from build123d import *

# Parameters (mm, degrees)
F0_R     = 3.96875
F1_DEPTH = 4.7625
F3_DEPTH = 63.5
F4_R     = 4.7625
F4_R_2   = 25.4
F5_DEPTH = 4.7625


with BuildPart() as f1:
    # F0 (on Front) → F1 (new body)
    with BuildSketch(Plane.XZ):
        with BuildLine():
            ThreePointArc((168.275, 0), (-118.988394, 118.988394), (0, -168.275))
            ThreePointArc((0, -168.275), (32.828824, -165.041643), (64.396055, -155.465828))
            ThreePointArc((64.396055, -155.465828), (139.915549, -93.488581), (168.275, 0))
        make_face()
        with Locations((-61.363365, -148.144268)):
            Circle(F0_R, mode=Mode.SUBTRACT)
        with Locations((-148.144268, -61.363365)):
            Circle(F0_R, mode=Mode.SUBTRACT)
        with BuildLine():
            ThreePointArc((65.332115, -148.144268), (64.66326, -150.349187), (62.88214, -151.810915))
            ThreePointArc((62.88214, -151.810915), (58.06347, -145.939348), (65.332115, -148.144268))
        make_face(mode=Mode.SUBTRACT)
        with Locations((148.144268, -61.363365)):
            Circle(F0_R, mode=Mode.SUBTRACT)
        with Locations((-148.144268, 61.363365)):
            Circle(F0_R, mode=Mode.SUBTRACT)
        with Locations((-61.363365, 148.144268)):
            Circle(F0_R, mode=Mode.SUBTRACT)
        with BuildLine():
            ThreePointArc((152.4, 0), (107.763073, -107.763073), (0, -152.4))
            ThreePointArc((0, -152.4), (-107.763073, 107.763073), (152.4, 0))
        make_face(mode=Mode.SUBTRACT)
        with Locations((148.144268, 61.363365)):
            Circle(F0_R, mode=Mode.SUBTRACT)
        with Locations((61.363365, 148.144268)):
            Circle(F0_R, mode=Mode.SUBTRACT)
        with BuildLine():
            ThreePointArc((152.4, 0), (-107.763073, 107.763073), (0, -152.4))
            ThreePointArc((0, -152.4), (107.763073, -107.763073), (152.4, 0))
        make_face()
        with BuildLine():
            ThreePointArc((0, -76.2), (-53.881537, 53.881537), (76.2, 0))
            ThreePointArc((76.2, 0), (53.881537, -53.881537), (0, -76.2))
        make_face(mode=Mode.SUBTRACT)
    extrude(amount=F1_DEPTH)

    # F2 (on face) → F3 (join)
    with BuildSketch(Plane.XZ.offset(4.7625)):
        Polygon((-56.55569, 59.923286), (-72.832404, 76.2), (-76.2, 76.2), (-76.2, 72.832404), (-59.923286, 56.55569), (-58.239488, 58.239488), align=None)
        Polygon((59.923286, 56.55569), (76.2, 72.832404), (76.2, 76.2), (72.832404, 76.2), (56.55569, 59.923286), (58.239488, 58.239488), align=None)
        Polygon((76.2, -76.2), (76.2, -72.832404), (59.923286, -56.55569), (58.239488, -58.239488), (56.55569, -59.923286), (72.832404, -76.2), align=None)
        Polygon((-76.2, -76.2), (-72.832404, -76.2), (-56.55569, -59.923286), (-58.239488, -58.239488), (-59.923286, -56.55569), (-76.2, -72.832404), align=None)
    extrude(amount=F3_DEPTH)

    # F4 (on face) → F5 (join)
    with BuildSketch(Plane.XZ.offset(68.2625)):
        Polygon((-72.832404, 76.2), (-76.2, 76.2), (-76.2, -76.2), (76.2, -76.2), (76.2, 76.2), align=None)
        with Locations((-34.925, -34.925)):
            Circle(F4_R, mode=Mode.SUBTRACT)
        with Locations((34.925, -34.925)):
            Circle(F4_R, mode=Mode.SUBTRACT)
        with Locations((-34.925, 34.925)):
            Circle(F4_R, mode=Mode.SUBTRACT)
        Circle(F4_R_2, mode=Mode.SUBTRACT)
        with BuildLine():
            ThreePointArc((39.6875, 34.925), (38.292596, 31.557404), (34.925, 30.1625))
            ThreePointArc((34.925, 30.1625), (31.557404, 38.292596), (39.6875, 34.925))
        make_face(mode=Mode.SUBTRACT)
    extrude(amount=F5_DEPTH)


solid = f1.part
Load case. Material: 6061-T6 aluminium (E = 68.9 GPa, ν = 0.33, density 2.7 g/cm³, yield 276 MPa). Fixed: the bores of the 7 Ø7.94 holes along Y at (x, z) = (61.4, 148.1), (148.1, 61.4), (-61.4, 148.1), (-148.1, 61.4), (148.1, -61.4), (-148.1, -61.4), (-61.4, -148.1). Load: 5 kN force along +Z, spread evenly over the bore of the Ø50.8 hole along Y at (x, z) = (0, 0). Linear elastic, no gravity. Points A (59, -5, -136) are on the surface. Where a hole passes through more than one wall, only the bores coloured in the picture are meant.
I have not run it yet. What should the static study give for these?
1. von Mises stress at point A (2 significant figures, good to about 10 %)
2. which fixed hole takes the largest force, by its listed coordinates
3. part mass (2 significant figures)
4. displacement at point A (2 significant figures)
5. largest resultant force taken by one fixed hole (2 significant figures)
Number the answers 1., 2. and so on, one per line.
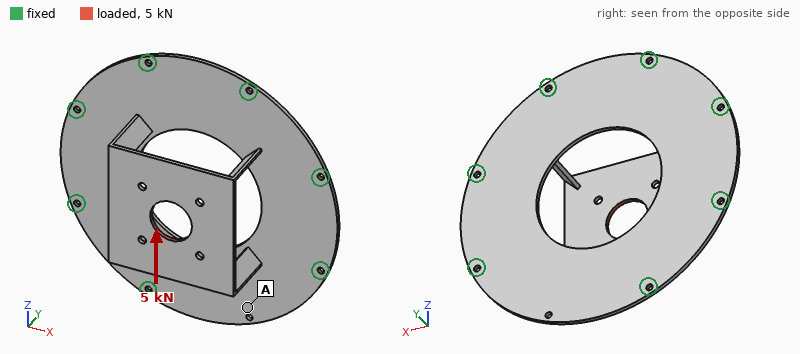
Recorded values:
1. 28 MPa
2. (-61.4, -148.1)
3. 1.3 kg
4. 0.88 mm
5. 1.2 kN
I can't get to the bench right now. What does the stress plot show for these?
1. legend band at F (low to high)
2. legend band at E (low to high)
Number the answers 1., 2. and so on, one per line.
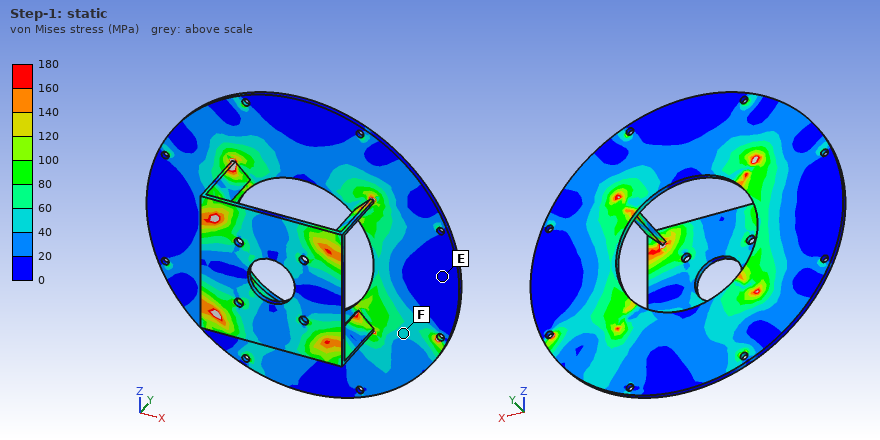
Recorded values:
1. 40 to 60 MPa
2. 0 to 20 MPa
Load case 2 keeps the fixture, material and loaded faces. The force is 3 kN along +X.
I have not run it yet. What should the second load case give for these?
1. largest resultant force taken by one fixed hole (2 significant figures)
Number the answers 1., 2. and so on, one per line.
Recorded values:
1. 660 N
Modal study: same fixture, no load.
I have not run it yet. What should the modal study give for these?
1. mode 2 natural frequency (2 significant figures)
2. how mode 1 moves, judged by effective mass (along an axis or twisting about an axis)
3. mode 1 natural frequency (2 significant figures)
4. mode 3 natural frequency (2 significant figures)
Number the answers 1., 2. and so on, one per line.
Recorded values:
1. 480 Hz
2. along Y
3. 380 Hz
4. 480 Hz
